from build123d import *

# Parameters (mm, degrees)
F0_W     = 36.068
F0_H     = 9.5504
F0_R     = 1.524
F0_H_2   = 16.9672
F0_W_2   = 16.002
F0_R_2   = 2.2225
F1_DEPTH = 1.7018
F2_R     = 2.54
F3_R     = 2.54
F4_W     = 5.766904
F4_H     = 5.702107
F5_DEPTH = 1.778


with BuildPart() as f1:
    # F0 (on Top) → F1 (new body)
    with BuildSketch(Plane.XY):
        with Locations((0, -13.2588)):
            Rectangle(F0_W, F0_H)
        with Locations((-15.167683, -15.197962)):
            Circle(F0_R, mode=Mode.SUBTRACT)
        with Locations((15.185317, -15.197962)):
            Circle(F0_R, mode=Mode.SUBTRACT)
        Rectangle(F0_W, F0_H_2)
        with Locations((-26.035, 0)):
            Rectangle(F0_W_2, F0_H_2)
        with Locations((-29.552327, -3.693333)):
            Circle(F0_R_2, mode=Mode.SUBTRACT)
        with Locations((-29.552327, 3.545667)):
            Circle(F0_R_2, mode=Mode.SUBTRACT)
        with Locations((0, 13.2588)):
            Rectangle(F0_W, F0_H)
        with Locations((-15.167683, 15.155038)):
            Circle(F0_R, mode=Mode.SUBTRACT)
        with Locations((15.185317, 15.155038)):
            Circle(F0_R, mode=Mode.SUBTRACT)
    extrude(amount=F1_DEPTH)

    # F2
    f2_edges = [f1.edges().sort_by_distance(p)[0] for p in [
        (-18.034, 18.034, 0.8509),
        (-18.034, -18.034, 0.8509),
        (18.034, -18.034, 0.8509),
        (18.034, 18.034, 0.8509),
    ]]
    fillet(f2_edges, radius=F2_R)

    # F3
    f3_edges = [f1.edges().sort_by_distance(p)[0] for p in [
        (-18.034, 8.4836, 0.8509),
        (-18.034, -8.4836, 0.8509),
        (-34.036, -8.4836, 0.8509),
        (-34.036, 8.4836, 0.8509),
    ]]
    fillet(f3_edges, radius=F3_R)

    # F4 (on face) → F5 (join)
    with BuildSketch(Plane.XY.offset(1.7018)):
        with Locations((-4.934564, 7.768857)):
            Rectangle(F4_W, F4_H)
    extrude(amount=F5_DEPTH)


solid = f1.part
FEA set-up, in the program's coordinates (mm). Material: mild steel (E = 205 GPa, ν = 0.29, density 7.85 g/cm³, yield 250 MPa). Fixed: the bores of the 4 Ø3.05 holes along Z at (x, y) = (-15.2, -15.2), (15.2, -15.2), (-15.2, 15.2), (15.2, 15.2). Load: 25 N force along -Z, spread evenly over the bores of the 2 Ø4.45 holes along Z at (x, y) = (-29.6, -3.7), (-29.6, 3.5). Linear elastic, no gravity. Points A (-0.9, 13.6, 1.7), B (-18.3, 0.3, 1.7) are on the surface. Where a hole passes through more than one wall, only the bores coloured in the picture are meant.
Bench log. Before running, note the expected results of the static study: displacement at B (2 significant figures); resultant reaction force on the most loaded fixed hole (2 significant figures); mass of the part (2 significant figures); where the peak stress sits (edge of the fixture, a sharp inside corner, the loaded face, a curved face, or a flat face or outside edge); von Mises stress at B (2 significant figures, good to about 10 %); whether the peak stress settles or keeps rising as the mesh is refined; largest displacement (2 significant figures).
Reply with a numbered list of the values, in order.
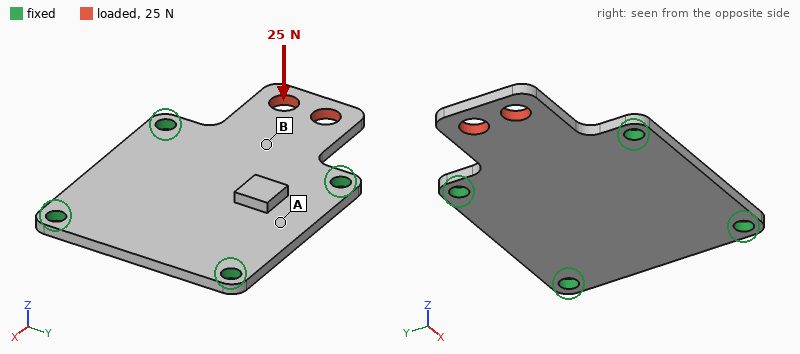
1. 7.3 µm
2. 16 N
3. 21 g
4. edge of the fixture
5. 28 MPa
6. keeps rising
7. 42 µm
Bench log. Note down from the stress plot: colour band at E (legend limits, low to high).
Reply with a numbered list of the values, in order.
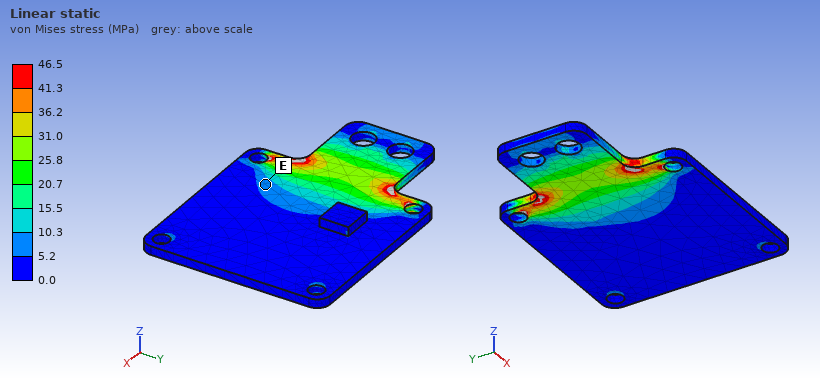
1. 5.2 to 10.3 MPa
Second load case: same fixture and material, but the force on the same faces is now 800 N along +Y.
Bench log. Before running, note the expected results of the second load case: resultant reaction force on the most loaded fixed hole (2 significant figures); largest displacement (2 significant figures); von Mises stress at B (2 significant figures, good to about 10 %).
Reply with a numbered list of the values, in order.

1. 520 N
2. 19 µm
3. 22 MPa
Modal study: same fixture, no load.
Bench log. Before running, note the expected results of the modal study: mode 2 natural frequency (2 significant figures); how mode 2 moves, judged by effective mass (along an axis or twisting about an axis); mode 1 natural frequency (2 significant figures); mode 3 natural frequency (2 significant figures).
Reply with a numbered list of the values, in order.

1. 6900 Hz
2. along Z
3. 3300 Hz
4. 10 kHz
